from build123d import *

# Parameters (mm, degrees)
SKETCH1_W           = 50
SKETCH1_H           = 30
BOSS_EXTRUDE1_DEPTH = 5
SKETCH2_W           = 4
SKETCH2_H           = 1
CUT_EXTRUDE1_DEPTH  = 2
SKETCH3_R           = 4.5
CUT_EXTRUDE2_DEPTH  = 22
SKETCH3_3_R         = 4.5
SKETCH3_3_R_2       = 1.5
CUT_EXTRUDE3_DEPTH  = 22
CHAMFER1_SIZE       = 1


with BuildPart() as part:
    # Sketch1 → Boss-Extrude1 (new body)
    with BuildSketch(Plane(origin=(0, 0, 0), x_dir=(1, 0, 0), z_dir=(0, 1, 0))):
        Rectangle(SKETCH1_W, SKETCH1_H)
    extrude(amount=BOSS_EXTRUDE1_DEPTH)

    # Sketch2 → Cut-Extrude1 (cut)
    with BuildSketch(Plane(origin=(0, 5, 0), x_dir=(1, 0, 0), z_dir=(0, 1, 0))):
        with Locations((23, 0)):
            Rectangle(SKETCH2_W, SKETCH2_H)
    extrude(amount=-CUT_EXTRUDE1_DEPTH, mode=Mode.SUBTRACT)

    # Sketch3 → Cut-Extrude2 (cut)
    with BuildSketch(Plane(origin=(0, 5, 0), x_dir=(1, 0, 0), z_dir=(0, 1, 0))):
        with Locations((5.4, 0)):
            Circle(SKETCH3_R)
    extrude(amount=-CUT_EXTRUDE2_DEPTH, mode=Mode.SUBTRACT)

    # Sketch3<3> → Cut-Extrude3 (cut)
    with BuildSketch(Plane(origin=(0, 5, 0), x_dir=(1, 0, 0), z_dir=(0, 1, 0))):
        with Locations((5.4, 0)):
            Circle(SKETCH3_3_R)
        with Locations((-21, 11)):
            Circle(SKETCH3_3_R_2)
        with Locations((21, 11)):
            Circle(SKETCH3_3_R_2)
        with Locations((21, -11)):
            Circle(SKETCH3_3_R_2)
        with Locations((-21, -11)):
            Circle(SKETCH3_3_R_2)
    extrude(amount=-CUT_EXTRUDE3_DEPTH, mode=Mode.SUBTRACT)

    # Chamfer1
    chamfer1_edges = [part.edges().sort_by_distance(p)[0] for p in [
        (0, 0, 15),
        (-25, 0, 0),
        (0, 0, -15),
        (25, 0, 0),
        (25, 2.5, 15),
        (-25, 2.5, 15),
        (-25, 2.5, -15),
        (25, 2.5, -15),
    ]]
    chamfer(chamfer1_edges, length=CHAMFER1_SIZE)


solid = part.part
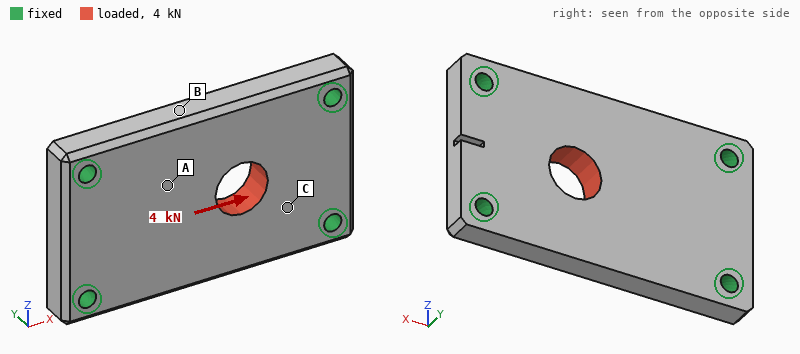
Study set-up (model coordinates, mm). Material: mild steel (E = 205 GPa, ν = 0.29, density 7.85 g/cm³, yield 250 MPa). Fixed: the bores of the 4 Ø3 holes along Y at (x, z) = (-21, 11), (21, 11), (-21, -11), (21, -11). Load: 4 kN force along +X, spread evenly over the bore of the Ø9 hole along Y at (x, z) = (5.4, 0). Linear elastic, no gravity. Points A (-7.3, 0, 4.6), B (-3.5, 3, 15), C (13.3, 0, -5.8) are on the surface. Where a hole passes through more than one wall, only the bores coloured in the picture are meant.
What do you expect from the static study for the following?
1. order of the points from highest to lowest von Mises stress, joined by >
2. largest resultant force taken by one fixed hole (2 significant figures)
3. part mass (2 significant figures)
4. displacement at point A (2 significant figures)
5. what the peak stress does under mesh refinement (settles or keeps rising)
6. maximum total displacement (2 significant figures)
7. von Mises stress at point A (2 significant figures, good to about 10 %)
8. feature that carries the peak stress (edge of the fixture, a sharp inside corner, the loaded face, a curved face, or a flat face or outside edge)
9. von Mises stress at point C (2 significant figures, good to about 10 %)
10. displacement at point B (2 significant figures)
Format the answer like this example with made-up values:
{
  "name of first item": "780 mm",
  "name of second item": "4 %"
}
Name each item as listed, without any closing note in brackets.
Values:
{
  "order of the points from highest to lowest von Mises stress, joined by >": "C > A > B",
  "largest resultant force taken by one fixed hole": "1.2 kN",
  "part mass": "55 g",
  "displacement at point A": "1.2 µm",
  "what the peak stress does under mesh refinement": "keeps rising",
  "maximum total displacement": "2.2 µm",
  "von Mises stress at point A": "16 MPa",
  "feature that carries the peak stress": "edge of the fixture",
  "von Mises stress at point C": "24 MPa",
  "displacement at point B": "0.99 µm"
}
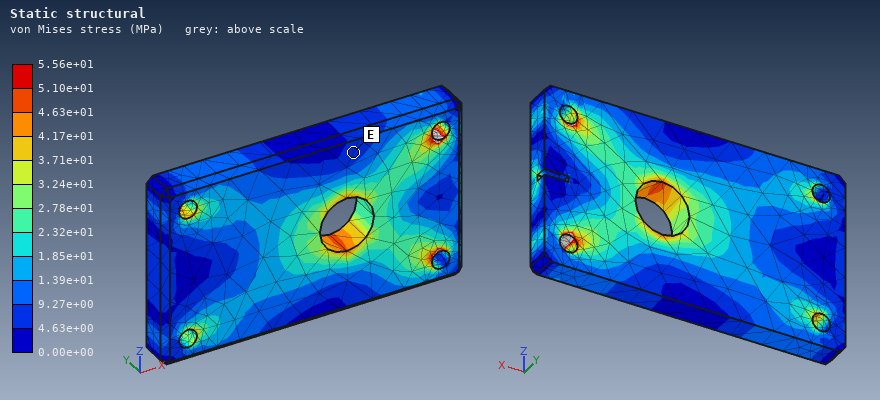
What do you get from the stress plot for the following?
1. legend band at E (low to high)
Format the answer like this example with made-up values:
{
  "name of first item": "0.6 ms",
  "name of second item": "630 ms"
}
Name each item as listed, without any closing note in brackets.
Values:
{
  "legend band at E": "4.63e+00 to 9.27e+00 MPa"
}
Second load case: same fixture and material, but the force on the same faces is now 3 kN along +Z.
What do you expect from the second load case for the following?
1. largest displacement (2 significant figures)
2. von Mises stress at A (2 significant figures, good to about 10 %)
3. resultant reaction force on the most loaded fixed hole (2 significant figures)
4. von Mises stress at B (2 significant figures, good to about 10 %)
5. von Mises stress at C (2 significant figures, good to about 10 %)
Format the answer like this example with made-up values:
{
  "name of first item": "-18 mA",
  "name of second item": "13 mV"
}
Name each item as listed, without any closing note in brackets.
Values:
{
  "largest displacement": "3.6 µm",
  "von Mises stress at A": "17 MPa",
  "resultant reaction force on the most loaded fixed hole": "1.1 kN",
  "von Mises stress at B": "13 MPa",
  "von Mises stress at C": "26 MPa"
}
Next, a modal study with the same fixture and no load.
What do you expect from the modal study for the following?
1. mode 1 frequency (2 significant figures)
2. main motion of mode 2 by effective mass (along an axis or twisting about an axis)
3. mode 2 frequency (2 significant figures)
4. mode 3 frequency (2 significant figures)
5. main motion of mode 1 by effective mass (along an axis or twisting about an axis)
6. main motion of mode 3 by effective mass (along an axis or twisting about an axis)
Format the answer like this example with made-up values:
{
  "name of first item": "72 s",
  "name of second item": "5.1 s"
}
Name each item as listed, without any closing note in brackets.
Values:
{
  "mode 1 frequency": "13 kHz",
  "main motion of mode 2 by effective mass": "twisting about X",
  "mode 2 frequency": "18 kHz",
  "mode 3 frequency": "30 kHz",
  "main motion of mode 1 by effective mass": "along Y",
  "main motion of mode 3 by effective mass": "twisting about Z"
}
